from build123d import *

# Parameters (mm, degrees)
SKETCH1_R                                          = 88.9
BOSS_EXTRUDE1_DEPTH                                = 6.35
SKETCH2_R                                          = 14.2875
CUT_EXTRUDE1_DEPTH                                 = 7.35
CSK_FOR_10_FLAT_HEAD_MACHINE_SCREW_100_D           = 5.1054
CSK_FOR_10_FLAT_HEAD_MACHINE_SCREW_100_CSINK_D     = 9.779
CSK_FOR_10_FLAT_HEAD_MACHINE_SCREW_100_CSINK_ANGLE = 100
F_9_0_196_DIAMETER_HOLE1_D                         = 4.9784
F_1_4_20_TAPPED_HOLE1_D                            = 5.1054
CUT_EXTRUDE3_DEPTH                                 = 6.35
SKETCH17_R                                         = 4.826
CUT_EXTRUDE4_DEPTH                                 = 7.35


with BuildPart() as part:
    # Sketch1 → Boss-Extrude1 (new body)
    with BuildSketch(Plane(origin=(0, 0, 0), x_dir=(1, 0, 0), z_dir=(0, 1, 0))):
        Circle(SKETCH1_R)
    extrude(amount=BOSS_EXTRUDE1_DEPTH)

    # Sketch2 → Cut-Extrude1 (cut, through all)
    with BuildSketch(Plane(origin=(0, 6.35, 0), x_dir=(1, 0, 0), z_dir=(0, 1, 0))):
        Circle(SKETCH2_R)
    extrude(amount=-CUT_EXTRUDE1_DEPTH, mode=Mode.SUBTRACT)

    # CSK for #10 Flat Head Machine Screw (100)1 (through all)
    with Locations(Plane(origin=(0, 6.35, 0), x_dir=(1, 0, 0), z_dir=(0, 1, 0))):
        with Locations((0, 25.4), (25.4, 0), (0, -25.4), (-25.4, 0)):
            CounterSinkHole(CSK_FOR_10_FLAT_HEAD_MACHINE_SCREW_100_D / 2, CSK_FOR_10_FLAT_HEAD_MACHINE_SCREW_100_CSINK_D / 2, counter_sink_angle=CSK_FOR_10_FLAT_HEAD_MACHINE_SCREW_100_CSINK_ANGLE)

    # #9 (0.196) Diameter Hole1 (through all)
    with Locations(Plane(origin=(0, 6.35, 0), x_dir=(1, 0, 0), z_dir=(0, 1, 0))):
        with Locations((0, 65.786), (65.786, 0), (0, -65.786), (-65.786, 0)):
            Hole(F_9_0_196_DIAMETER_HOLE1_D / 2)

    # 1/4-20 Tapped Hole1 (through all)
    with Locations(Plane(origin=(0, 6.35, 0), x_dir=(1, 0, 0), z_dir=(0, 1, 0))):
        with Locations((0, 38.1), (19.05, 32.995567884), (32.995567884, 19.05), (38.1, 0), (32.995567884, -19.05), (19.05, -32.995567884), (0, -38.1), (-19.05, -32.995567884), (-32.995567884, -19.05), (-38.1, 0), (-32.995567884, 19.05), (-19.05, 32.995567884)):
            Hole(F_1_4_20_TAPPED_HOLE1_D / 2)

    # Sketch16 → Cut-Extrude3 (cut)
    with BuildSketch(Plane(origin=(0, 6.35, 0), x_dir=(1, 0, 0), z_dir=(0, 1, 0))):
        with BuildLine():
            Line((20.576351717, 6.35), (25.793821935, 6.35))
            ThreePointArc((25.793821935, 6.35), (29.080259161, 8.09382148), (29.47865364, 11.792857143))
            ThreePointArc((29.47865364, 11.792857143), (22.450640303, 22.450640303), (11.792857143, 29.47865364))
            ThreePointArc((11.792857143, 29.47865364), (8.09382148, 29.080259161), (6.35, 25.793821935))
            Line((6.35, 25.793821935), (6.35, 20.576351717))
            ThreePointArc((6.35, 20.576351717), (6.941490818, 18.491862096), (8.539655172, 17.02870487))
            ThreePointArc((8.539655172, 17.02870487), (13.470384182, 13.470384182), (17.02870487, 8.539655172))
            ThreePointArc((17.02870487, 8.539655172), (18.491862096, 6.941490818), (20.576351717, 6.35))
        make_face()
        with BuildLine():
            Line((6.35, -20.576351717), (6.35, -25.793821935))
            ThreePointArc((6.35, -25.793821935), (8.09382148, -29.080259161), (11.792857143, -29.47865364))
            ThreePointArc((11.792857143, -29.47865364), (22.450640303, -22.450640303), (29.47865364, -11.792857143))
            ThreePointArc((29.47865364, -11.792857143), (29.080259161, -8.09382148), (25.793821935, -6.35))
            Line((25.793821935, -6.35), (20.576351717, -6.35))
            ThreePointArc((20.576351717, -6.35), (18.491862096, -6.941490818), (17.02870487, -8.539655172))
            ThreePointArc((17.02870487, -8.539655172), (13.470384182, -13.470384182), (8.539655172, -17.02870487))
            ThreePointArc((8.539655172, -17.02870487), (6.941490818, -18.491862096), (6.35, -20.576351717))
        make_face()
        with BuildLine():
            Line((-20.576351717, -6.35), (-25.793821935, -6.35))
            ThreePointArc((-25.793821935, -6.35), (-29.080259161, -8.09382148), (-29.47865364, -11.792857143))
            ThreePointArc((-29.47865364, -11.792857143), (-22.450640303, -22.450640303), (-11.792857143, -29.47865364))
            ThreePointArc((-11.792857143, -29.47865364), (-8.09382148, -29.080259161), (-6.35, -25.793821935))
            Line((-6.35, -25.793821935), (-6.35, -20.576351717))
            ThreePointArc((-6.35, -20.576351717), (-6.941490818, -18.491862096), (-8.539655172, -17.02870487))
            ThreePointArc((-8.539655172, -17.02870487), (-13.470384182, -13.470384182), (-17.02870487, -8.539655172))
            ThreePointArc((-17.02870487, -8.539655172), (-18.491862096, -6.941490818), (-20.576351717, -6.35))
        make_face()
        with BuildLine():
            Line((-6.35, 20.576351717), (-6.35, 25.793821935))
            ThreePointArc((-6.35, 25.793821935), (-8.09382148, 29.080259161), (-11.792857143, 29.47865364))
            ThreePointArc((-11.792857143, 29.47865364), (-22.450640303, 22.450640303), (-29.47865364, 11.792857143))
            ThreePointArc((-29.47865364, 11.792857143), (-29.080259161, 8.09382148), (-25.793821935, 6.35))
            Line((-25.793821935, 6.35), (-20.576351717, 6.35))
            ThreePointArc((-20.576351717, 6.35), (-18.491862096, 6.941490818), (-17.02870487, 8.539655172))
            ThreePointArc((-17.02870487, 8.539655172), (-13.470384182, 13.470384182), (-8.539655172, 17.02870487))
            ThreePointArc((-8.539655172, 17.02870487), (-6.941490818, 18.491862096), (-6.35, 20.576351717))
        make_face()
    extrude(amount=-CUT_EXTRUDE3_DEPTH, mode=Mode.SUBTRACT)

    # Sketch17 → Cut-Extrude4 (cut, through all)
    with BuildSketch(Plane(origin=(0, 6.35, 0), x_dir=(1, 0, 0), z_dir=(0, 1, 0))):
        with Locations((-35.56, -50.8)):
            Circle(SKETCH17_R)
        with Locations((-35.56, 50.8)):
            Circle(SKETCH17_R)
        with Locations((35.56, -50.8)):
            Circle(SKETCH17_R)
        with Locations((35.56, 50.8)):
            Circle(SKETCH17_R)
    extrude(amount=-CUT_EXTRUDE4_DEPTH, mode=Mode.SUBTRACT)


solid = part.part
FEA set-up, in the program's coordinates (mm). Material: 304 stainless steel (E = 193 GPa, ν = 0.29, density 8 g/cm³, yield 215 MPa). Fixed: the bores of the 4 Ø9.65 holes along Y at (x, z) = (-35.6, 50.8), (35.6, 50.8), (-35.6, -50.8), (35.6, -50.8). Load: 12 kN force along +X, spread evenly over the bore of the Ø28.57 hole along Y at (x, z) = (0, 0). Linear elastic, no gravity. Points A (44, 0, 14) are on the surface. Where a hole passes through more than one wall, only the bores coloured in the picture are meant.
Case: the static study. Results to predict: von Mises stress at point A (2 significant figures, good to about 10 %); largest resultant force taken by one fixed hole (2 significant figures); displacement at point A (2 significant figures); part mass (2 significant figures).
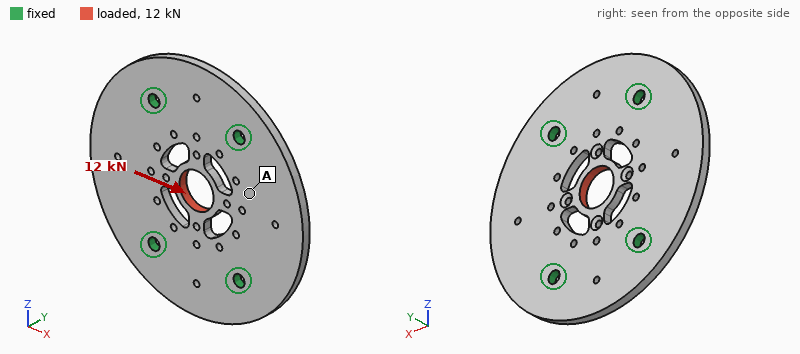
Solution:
20 MPa
3.0 kN
4.6 µm
1.1 kg
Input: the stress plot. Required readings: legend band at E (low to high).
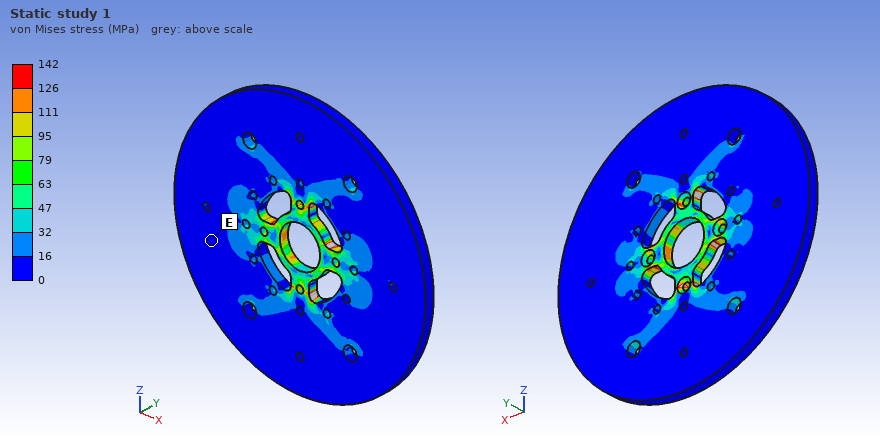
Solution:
0 to 16 MPa
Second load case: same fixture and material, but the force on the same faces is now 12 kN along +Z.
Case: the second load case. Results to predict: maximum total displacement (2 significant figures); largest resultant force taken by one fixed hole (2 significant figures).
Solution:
24 µm
3.1 kN
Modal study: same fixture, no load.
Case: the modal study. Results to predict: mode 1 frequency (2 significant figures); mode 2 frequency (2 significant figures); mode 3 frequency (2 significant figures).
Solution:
1700 Hz
1700 Hz
3300 Hz
